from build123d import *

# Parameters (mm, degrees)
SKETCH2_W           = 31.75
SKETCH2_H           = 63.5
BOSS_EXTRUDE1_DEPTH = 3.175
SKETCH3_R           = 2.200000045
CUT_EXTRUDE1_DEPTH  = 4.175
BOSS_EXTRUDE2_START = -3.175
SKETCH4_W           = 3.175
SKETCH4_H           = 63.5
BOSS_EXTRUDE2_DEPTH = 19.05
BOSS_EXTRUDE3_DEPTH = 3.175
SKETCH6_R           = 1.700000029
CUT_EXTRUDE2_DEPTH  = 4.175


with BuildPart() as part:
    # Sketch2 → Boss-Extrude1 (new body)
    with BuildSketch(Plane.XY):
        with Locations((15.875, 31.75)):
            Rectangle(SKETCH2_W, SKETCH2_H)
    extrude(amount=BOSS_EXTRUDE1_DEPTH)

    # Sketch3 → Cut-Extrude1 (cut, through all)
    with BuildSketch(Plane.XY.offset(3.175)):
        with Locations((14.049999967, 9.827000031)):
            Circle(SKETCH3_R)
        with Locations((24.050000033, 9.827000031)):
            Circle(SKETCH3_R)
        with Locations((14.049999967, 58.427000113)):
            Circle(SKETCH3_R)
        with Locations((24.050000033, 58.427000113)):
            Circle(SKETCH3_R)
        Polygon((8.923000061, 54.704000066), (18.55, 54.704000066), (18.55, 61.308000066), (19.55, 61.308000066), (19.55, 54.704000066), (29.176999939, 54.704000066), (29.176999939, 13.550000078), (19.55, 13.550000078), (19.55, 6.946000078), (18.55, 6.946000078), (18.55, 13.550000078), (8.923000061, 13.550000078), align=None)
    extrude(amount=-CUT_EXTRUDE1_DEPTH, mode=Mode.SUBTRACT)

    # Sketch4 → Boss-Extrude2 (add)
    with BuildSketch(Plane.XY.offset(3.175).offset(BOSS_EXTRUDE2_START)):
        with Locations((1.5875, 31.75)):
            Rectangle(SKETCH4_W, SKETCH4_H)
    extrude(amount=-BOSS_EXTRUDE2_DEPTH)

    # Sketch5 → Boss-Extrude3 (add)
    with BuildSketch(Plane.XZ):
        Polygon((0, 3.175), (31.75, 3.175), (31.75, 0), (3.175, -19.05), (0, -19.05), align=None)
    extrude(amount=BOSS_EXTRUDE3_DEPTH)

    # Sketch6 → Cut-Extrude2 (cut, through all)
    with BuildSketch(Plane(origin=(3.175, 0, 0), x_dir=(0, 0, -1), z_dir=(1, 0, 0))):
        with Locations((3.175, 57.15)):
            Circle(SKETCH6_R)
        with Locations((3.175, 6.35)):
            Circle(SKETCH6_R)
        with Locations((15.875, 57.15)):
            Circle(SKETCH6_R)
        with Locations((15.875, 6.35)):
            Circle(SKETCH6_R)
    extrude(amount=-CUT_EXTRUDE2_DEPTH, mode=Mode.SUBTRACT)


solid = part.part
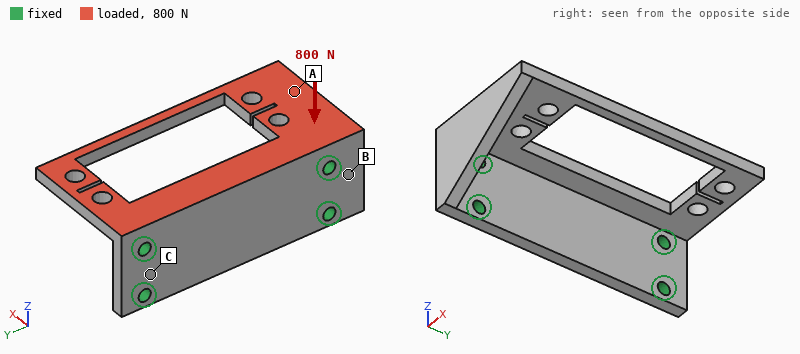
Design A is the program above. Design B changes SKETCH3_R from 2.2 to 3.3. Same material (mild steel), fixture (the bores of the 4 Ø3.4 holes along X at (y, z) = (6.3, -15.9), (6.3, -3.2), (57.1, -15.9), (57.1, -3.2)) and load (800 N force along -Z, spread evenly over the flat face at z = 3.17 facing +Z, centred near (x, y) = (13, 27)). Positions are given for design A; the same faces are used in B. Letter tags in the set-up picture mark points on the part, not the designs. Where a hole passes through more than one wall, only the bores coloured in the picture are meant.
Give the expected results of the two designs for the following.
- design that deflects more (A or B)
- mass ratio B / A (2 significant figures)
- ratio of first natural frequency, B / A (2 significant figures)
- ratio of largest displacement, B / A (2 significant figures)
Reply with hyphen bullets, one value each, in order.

- B
- 0.97
- 0.95
- 1.1
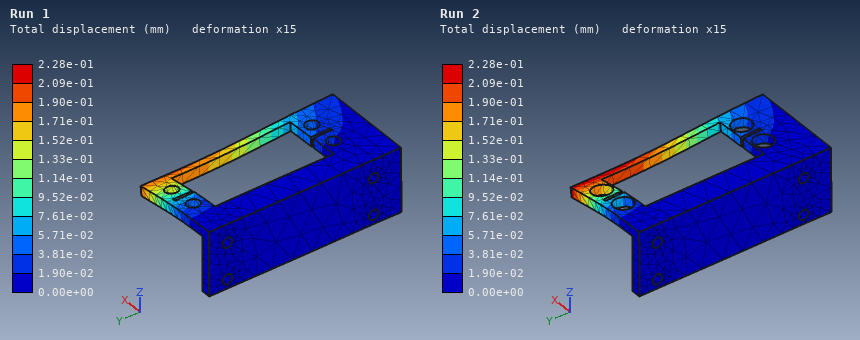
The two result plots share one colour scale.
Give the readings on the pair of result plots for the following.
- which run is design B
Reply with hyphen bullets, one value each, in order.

- Run 2
